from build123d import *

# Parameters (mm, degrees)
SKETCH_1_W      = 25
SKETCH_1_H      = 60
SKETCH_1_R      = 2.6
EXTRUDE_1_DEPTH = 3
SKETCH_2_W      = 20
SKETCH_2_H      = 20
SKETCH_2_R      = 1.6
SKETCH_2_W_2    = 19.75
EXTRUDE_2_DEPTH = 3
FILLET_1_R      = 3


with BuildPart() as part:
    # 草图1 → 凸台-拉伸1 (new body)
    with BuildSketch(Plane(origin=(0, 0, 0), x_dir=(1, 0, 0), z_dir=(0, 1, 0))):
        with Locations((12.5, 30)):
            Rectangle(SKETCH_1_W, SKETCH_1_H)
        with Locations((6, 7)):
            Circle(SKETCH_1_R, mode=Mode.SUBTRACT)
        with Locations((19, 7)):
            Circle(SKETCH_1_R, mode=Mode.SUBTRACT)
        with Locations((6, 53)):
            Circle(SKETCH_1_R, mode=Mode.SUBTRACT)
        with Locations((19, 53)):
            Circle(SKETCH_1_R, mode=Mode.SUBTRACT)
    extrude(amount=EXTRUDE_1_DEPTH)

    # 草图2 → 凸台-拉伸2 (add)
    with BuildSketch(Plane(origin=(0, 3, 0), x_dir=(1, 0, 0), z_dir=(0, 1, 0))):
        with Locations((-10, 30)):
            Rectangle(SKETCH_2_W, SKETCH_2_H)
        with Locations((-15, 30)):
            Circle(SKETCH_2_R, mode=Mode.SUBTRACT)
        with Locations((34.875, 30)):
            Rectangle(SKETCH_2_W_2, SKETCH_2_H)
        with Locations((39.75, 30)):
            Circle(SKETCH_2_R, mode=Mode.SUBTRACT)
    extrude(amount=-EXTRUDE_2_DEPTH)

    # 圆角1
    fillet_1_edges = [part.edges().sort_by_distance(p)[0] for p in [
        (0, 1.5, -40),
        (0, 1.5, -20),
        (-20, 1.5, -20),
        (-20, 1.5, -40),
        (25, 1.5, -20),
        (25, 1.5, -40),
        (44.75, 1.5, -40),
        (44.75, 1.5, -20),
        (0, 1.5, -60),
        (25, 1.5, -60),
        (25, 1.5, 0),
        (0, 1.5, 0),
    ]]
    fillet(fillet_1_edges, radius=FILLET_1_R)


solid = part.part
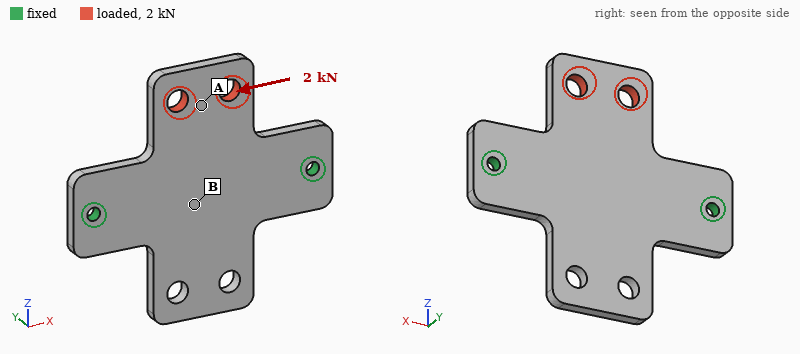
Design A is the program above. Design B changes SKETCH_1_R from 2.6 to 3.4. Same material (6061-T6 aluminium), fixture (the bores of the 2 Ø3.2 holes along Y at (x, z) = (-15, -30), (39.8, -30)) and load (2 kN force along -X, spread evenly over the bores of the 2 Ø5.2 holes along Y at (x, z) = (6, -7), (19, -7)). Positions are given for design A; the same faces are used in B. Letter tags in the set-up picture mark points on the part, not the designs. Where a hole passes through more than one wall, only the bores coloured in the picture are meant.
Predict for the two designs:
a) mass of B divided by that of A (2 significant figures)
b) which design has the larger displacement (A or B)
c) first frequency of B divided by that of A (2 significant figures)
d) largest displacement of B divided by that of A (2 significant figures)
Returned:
0.97
B
1.0
1.1
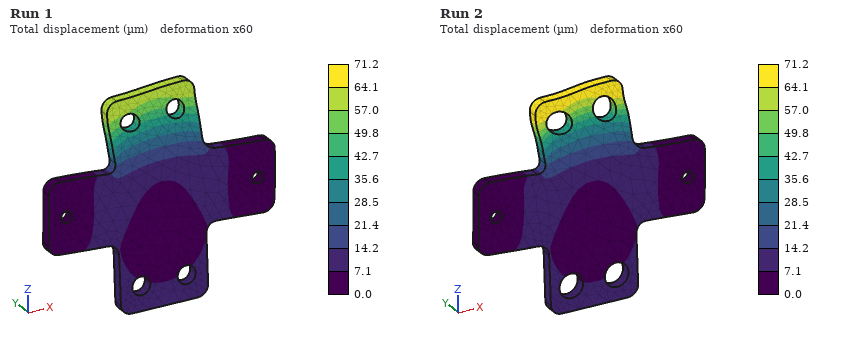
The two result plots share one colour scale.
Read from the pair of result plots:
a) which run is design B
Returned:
Run 2
